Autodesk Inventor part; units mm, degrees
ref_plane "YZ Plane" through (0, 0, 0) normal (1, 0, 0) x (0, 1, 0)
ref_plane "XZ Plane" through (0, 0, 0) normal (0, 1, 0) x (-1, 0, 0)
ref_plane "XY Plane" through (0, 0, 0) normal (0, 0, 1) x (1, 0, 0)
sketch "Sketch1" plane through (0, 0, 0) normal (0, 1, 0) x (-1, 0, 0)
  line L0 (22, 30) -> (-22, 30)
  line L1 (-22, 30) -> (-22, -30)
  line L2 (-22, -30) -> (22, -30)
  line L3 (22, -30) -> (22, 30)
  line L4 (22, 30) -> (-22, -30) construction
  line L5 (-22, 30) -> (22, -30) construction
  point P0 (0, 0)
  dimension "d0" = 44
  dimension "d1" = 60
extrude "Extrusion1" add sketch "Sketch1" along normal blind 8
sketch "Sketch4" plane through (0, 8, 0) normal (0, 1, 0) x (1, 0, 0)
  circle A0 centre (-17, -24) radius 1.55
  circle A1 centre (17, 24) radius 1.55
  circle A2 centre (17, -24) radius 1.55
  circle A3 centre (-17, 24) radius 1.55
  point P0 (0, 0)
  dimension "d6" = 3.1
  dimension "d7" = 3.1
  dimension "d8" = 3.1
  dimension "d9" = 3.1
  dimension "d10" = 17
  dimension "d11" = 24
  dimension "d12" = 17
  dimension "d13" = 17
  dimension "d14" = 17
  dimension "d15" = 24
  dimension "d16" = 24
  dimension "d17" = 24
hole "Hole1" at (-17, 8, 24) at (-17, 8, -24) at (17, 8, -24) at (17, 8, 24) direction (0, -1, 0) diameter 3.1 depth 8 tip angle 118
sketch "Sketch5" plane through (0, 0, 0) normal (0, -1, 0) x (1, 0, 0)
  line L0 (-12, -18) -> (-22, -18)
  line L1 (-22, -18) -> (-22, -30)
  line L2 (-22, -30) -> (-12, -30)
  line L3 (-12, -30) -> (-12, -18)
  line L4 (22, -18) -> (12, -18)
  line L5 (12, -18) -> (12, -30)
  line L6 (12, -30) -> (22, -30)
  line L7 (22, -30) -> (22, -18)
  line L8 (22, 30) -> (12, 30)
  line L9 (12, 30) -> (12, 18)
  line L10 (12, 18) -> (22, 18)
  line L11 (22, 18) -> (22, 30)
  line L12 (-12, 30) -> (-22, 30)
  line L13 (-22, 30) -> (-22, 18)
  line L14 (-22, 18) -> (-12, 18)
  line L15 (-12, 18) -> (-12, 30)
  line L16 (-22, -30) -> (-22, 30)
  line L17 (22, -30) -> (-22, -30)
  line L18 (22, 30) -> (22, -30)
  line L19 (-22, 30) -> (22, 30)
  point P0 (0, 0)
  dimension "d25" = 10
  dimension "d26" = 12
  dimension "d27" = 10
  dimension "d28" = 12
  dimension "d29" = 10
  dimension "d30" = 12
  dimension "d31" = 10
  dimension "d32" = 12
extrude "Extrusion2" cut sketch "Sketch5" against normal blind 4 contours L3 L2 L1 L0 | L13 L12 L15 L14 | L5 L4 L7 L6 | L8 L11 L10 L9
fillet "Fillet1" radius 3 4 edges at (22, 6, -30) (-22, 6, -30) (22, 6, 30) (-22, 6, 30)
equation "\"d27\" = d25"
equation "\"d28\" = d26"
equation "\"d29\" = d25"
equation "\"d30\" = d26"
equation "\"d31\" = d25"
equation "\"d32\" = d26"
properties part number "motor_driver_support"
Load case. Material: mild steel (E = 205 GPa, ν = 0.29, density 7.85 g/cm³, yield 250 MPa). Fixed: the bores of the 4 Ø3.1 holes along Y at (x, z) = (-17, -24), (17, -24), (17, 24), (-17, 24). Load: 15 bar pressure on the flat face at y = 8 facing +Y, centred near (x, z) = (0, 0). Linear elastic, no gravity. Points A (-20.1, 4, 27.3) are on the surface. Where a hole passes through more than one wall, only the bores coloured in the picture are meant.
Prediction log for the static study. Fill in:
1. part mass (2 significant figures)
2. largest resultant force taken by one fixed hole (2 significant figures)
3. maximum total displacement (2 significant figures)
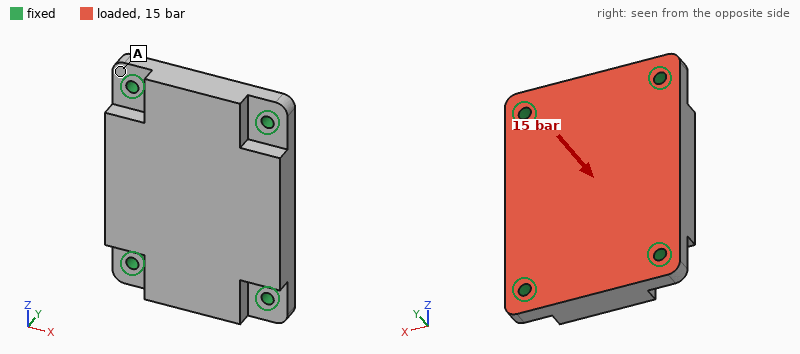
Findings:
150 g
1.1 kN
8.2 µm
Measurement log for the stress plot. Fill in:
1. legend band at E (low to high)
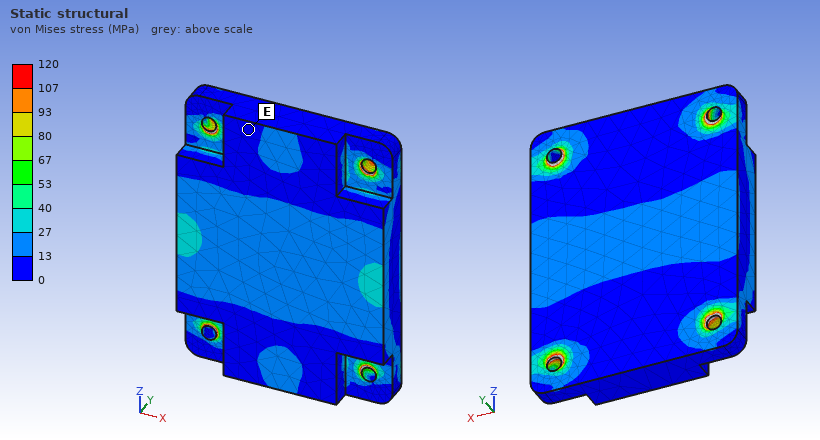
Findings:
0 to 13 MPa
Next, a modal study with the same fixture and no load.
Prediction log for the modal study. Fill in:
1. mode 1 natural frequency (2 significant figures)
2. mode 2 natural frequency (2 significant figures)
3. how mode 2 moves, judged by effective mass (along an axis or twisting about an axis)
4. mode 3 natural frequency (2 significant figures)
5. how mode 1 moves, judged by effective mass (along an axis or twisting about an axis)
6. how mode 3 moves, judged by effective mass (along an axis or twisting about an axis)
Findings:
9700 Hz
14 kHz
twisting about Z
19 kHz
along Y
twisting about X
